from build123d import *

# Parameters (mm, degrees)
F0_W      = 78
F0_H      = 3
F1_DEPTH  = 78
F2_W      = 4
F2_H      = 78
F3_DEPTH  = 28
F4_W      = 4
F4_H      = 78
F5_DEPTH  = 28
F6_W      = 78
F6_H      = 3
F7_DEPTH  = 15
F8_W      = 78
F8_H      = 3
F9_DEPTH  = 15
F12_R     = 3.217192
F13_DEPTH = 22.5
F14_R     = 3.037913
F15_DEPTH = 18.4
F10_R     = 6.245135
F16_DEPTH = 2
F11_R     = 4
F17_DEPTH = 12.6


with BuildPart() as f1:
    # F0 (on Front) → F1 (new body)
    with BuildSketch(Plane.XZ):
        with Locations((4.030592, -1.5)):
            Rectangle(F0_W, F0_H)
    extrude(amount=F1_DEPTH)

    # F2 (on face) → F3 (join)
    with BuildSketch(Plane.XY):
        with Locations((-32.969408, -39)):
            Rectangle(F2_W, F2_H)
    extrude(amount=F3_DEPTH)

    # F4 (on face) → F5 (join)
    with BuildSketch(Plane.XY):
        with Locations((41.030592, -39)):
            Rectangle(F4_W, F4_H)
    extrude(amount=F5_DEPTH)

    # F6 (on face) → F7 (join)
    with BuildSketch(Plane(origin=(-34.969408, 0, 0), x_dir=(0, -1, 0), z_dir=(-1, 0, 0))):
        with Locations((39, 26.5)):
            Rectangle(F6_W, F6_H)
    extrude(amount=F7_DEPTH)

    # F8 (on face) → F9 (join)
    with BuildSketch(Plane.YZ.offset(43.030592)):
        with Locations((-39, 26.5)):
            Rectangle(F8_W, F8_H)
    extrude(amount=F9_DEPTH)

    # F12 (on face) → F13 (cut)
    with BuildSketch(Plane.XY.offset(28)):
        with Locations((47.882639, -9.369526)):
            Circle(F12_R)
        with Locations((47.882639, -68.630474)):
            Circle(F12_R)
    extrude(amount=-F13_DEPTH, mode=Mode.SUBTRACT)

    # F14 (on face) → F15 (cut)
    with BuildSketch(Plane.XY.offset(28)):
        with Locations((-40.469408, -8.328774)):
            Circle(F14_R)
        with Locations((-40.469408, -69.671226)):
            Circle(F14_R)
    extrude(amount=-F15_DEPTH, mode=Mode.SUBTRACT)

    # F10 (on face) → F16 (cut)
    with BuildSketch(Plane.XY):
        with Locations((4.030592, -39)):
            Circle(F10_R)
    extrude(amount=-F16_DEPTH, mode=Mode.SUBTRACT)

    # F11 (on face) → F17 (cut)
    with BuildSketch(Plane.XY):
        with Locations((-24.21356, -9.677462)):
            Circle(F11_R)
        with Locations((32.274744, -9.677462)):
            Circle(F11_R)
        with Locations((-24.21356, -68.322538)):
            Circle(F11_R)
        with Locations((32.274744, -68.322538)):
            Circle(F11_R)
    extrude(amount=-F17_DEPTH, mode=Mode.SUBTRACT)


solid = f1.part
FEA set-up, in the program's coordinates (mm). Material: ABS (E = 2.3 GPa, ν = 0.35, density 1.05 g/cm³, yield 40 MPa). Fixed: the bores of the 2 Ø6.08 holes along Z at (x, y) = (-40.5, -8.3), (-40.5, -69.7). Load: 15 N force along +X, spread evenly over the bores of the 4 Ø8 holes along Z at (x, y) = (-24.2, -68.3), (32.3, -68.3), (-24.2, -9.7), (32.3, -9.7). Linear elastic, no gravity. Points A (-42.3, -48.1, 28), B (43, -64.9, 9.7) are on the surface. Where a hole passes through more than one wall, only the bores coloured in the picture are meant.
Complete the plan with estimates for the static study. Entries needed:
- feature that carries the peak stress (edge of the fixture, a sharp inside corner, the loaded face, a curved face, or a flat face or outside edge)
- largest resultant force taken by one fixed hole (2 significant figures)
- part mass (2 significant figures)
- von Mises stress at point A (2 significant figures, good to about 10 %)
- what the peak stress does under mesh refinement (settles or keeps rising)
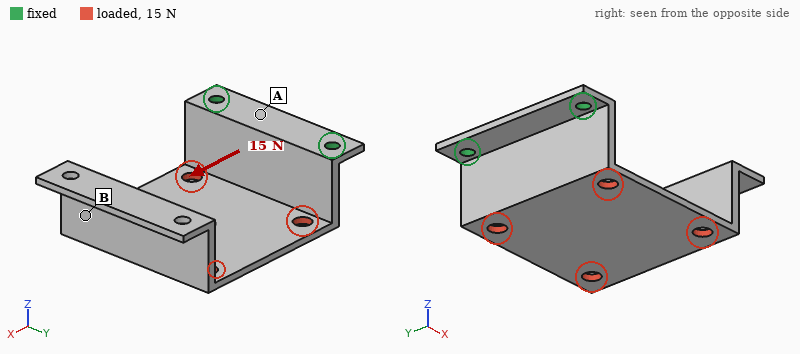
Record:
edge of the fixture
7.5 N
44 g
1.2 MPa
keeps rising
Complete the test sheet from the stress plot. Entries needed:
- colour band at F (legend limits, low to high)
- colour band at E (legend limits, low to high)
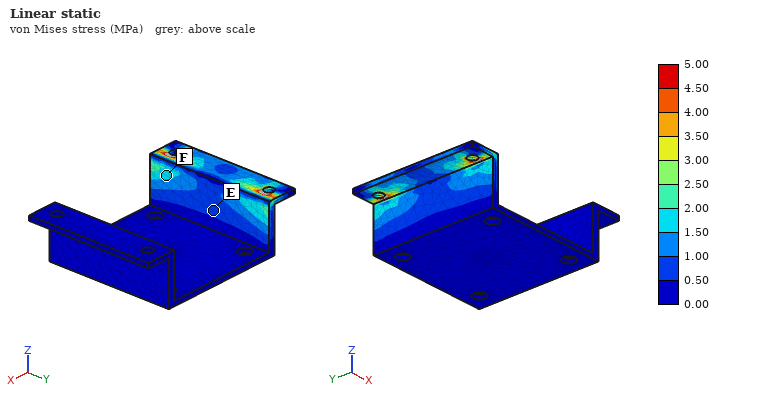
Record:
1.50 to 2.00 MPa
0.50 to 1.00 MPa
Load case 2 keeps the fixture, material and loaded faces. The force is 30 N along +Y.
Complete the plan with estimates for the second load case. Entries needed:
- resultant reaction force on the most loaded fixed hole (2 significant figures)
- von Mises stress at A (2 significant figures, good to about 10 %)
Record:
29 N
0.52 MPa
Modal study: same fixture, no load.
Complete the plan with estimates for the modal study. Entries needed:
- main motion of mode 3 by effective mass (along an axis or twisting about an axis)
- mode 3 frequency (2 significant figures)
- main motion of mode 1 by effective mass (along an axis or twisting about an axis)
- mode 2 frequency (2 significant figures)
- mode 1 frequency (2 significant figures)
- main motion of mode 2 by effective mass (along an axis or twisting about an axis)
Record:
along X
170 Hz
along Z
110 Hz
46 Hz
along Y
